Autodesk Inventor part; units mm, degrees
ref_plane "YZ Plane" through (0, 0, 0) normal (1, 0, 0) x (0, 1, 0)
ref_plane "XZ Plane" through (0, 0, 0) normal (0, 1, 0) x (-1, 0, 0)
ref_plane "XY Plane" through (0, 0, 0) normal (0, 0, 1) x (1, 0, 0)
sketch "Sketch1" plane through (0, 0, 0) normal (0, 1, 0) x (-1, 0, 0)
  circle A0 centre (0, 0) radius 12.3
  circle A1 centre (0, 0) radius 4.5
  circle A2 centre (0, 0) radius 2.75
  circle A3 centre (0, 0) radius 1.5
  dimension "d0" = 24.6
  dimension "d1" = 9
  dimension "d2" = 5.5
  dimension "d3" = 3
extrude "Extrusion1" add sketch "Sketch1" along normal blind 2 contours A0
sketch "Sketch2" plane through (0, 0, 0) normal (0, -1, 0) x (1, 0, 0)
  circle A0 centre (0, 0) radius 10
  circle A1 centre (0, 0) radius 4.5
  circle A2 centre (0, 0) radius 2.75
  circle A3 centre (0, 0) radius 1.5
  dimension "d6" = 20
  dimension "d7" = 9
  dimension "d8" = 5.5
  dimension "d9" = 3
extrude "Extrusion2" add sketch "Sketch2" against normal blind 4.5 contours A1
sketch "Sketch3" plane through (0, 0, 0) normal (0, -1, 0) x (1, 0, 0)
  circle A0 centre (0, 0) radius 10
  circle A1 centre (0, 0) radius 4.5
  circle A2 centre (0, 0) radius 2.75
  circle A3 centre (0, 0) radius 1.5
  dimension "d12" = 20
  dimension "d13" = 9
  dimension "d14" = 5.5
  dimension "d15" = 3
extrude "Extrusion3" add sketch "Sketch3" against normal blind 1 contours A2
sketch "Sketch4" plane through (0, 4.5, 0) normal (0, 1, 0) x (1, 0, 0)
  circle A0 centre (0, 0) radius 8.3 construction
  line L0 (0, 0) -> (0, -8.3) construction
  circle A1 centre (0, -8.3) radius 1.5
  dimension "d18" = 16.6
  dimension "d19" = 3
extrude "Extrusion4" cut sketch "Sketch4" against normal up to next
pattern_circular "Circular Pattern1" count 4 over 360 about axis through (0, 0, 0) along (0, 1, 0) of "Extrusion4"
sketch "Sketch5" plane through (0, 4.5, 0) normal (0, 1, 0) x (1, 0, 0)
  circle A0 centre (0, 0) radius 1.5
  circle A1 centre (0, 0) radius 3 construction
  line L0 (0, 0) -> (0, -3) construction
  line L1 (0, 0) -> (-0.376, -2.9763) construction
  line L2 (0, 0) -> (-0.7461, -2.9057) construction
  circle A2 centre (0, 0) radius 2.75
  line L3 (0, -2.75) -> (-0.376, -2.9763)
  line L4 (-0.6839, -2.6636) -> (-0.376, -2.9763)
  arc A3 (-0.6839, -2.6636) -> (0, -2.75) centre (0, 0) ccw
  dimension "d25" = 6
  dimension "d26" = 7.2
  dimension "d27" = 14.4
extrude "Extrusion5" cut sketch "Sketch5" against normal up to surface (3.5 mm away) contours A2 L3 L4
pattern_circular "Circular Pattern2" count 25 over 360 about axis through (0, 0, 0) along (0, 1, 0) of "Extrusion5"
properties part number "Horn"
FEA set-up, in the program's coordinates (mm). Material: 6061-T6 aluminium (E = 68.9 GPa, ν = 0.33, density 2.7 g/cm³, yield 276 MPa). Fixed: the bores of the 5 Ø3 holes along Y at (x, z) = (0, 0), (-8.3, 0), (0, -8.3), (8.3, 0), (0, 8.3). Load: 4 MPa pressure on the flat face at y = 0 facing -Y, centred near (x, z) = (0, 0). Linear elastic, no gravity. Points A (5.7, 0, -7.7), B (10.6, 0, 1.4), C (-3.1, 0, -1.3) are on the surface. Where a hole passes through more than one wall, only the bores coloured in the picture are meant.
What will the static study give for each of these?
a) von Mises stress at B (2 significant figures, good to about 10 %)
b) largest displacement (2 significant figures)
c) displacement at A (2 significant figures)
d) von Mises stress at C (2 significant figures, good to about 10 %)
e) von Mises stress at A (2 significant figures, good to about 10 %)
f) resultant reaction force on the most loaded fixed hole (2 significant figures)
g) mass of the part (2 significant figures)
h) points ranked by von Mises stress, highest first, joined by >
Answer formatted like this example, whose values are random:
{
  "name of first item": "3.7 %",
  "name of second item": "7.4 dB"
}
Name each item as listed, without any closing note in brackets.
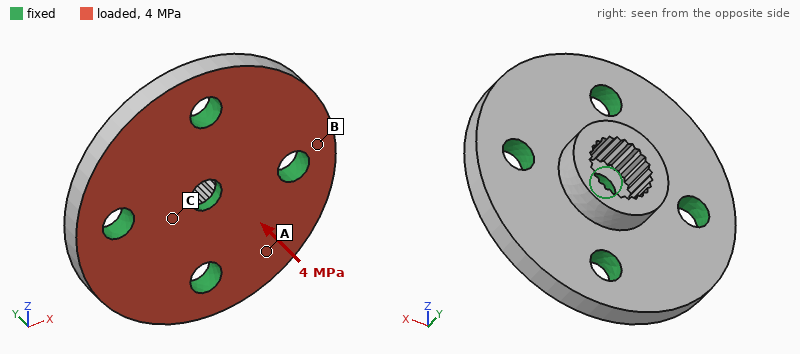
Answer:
{
  "von Mises stress at B": "43 MPa",
  "largest displacement": "14 µm",
  "displacement at A": "7.7 µm",
  "von Mises stress at C": "13 MPa",
  "von Mises stress at A": "26 MPa",
  "resultant reaction force on the most loaded fixed hole": "400 N",
  "mass of the part": "2.6 g",
  "points ranked by von Mises stress, highest first, joined by >": "B > A > C"
}
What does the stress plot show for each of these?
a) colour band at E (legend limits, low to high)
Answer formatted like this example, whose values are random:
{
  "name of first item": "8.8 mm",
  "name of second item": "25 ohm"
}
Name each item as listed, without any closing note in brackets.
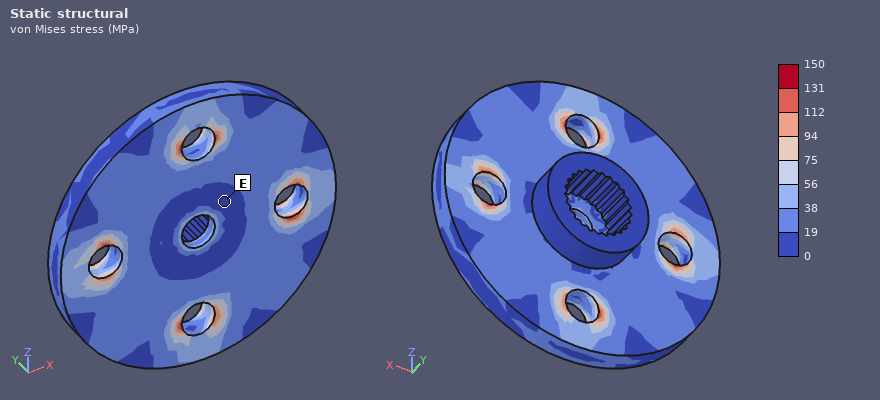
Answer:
{
  "colour band at E": "0 to 19 MPa"
}
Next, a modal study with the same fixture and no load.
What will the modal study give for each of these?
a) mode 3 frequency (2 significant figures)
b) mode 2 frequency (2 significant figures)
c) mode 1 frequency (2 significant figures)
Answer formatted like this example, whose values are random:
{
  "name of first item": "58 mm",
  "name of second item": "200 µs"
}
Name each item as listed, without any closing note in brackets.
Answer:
{
  "mode 3 frequency": "48 kHz",
  "mode 2 frequency": "48 kHz",
  "mode 1 frequency": "47 kHz"
}
